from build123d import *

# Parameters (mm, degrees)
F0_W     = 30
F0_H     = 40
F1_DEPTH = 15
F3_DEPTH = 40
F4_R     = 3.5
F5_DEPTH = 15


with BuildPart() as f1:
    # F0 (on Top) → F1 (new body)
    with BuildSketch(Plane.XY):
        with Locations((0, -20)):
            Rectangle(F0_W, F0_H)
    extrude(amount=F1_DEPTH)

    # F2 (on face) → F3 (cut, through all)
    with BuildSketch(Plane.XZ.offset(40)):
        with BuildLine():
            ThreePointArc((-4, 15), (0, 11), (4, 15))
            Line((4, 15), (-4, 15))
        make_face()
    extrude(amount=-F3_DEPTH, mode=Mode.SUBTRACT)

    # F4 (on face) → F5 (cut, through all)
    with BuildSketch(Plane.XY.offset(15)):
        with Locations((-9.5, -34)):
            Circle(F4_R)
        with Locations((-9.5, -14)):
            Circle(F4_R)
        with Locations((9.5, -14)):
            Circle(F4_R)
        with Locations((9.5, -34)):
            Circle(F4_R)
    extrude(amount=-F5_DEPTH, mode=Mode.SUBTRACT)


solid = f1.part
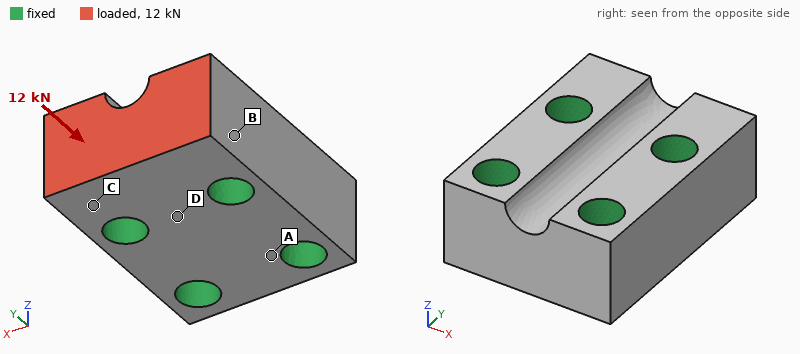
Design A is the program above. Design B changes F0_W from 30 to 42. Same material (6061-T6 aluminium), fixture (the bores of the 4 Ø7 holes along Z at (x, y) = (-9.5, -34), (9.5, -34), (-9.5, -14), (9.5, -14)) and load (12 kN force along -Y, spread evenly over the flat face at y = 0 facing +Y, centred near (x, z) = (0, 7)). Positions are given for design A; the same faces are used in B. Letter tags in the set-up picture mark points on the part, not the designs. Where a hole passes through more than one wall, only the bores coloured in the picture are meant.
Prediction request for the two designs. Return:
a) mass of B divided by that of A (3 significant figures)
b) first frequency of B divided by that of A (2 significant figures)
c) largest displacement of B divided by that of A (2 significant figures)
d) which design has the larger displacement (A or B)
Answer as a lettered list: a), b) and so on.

a) 1.49
b) 0.89
c) 1.2
d) B
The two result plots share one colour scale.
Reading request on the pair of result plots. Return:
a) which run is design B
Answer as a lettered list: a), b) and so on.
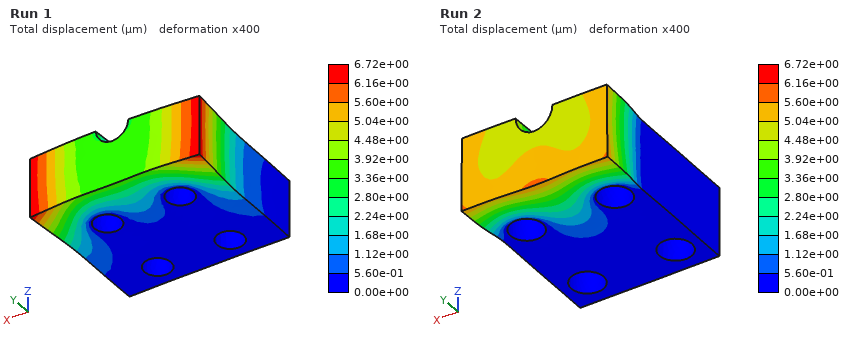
a) Run 1
